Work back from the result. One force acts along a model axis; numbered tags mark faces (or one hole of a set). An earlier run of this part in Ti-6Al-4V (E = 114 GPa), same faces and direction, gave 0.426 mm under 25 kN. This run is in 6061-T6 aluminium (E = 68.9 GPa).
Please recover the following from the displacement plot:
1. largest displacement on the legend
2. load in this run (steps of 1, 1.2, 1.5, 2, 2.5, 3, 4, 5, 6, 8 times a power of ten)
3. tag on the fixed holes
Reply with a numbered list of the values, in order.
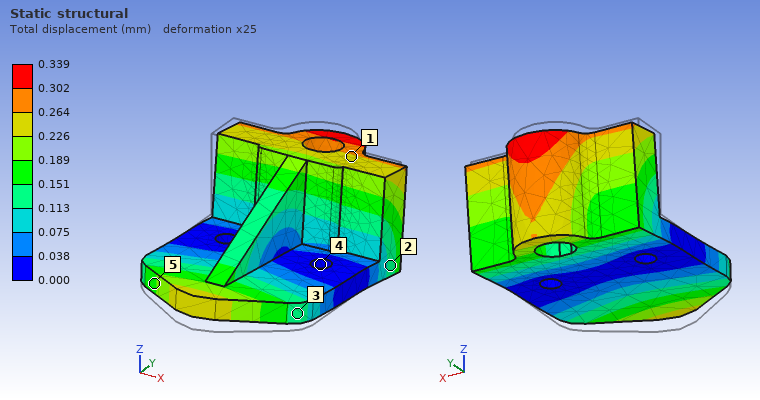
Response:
1. 0.339 mm
2. 12 kN
3. 4
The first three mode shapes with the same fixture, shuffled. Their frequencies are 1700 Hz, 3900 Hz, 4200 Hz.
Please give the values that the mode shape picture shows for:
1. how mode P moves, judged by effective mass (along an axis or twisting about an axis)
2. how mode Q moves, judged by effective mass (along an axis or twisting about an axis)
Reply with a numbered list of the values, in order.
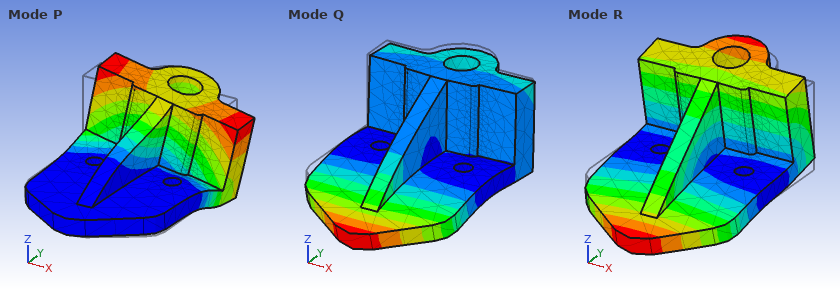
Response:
1. along X
2. along Z
